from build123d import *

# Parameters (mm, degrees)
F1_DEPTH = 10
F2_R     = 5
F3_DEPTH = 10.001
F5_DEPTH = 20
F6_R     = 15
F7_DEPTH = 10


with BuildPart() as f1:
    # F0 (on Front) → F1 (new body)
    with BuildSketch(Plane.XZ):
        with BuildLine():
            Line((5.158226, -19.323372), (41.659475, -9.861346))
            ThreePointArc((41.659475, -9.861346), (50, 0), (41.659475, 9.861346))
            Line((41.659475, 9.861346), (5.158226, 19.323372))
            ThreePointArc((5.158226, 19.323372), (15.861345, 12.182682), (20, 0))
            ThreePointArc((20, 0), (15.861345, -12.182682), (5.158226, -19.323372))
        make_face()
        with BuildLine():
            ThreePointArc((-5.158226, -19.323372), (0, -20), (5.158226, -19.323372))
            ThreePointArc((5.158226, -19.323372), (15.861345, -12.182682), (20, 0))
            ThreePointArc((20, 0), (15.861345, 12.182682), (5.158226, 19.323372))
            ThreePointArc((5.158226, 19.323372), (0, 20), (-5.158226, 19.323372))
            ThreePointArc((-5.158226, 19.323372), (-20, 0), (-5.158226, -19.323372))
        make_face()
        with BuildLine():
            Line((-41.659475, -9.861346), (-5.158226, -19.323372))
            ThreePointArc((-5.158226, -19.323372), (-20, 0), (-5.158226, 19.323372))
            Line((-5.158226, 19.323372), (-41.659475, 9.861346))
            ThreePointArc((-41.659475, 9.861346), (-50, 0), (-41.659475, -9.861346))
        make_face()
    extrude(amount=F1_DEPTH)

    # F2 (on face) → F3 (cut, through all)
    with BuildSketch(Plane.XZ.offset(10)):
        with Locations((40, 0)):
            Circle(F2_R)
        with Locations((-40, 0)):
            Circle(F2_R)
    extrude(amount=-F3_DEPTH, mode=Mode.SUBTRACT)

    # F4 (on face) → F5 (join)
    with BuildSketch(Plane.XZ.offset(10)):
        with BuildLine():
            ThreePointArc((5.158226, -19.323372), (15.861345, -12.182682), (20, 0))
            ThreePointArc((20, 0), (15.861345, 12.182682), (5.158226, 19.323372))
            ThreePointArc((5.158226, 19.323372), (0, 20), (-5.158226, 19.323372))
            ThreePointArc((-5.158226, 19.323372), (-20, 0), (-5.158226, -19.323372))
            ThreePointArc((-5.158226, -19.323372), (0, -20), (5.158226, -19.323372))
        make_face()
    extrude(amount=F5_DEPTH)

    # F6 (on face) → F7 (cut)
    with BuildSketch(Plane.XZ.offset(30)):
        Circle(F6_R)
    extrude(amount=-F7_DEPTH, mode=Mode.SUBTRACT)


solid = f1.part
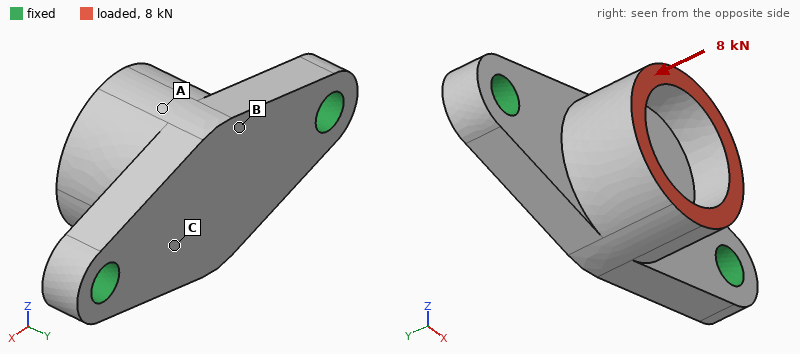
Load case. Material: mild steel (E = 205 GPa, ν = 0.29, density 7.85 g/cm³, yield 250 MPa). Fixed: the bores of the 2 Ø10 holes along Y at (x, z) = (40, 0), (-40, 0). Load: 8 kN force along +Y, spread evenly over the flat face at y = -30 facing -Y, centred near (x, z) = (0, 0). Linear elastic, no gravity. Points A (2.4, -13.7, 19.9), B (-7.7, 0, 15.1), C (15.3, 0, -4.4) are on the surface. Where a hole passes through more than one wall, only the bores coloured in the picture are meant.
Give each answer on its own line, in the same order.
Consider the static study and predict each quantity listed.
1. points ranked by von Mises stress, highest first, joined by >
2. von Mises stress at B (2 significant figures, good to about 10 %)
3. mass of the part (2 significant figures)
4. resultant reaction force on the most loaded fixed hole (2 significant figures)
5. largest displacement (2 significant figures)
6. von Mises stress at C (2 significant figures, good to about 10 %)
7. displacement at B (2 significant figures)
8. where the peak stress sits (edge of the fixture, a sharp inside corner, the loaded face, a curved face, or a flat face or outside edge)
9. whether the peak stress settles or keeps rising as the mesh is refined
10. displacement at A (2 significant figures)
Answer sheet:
C > B > A
23 MPa
350 g
4.3 kN
19 µm
42 MPa
16 µm
edge of the fixture
keeps rising
17 µm
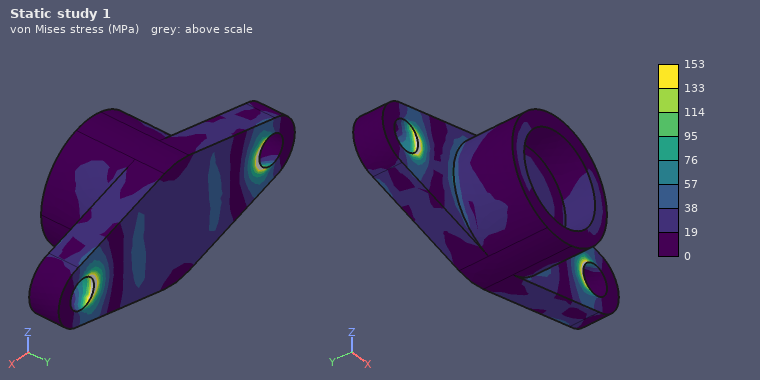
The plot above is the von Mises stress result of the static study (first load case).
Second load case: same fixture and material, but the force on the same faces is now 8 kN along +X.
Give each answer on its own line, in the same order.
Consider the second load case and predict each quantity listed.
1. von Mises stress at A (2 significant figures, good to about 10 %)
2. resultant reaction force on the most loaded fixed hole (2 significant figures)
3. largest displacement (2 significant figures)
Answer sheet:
11 MPa
5.3 kN
26 µm
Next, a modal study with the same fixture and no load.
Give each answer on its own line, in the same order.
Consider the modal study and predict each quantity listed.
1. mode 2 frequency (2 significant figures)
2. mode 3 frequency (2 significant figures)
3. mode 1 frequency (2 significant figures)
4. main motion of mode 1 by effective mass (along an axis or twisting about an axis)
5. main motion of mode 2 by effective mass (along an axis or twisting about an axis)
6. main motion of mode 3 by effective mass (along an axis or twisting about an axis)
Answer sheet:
6900 Hz
11 kHz
4800 Hz
along Z
along Y
along Z
